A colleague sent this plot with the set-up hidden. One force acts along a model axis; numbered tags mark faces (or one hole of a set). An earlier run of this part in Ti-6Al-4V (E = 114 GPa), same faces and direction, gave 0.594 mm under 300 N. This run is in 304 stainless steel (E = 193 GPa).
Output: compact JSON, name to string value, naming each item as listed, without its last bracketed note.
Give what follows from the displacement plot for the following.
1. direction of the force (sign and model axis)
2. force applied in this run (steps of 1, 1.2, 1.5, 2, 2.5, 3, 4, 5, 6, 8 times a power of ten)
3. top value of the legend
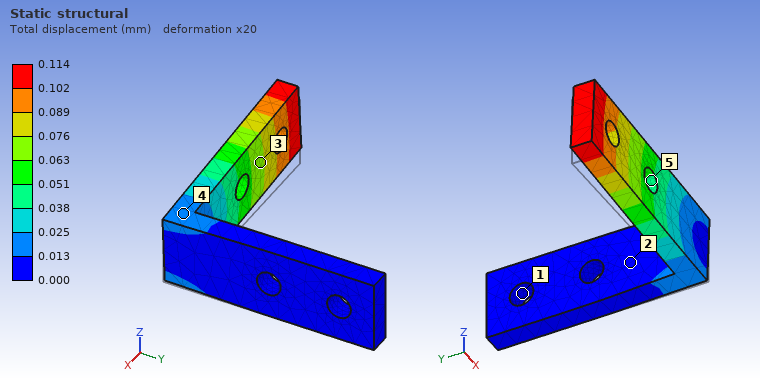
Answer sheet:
{"direction of the force": "+Z", "force applied in this run": "100 N", "top value of the legend": "0.114 mm"}
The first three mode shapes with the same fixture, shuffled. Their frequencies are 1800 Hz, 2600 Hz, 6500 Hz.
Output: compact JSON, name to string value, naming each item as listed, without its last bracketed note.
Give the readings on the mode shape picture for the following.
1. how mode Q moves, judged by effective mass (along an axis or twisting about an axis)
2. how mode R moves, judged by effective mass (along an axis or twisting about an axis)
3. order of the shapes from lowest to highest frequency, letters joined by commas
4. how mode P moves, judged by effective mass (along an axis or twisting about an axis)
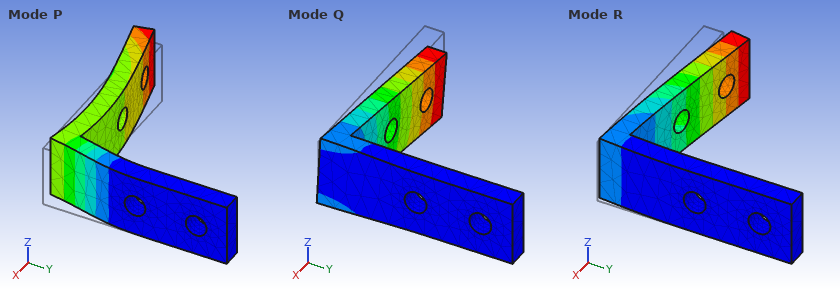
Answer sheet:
{"how mode Q moves, judged by effective mass": "along Z", "how mode R moves, judged by effective mass": "along Y", "order of the shapes from lowest to highest frequency, letters joined by commas": "R, Q, P", "how mode P moves, judged by effective mass": "along X"}
